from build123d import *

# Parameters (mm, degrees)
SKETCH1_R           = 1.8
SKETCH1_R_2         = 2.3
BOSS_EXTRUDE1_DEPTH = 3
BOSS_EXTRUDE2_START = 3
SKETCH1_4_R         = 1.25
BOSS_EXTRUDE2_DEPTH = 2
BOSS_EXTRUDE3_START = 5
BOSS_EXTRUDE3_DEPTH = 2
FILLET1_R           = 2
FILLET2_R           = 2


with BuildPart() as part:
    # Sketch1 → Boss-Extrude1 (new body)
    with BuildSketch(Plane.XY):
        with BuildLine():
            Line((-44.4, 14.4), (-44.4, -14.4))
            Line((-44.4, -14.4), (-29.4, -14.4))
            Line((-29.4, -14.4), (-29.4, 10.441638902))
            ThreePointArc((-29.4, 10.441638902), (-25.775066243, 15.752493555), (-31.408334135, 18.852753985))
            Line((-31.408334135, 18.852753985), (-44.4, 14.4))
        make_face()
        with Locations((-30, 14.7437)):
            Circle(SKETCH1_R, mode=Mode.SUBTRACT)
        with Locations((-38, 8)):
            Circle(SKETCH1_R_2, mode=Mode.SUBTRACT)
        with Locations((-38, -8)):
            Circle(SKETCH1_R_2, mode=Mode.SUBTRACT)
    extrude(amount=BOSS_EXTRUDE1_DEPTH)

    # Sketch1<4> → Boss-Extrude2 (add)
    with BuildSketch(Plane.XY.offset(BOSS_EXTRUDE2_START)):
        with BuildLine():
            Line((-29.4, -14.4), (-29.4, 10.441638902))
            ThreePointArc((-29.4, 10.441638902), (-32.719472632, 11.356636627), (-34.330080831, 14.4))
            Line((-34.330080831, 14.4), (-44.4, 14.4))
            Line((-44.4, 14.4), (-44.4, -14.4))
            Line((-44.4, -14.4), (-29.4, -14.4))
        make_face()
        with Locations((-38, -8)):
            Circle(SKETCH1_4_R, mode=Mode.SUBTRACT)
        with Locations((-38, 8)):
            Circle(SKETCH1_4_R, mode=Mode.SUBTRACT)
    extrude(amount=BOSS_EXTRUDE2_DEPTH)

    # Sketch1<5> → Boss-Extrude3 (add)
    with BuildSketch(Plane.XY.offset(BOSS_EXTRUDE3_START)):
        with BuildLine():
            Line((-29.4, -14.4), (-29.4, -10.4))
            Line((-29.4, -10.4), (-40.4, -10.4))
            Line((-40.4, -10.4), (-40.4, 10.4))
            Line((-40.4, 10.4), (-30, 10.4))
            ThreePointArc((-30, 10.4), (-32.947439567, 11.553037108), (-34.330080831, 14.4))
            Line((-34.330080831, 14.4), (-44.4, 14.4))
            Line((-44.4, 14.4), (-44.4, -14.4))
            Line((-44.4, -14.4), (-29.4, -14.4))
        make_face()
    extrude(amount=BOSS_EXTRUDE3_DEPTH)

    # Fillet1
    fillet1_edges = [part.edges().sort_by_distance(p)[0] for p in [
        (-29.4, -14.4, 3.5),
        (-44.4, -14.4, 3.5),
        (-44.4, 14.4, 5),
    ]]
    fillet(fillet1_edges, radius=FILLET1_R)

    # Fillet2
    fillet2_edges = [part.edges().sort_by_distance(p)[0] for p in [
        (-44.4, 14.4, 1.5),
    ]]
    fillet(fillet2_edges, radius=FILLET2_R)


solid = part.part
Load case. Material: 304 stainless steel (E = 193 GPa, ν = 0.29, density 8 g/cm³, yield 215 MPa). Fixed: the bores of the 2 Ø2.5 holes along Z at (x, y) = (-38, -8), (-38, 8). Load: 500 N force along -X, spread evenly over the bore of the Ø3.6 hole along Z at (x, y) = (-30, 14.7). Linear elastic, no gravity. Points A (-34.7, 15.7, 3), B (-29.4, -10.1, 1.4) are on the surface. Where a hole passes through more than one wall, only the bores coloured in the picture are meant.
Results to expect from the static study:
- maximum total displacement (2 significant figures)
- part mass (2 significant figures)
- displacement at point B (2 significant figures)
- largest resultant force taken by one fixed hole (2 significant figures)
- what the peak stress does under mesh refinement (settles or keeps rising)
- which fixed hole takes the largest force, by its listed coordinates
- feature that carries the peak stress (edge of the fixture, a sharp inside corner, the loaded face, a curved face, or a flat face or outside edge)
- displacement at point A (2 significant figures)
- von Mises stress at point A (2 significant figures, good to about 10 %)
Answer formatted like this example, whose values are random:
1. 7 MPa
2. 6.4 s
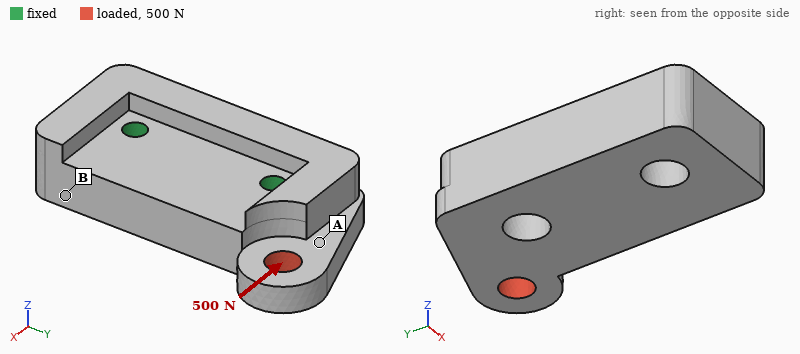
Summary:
1. 9.6 µm
2. 20 g
3. 1.9 µm
4. 670 N
5. keeps rising
6. (-38, 8)
7. edge of the fixture
8. 3.9 µm
9. 24 MPa
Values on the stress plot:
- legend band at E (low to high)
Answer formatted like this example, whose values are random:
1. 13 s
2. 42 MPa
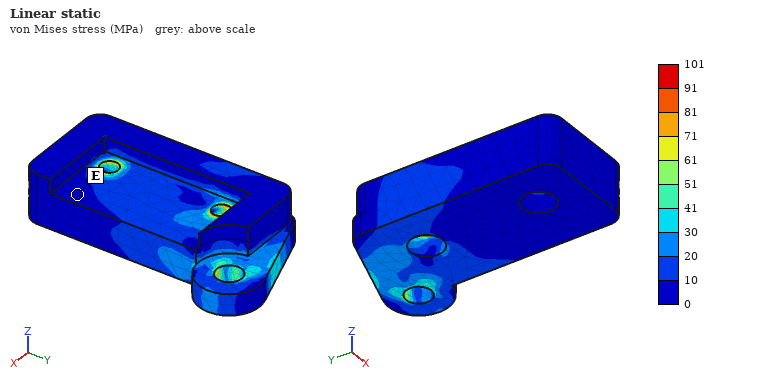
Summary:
1. 0 to 10 MPa
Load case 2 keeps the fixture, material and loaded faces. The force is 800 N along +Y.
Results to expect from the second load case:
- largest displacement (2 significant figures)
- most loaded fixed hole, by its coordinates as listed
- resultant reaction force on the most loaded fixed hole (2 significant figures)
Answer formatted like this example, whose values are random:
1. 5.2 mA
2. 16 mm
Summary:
1. 9.4 µm
2. (-38, 8)
3. 590 N
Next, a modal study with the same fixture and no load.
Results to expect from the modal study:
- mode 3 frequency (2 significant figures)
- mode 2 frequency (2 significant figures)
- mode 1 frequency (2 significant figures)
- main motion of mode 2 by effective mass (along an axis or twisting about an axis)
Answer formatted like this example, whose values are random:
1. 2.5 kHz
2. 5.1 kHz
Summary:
1. 29 kHz
2. 21 kHz
3. 13 kHz
4. twisting about X
